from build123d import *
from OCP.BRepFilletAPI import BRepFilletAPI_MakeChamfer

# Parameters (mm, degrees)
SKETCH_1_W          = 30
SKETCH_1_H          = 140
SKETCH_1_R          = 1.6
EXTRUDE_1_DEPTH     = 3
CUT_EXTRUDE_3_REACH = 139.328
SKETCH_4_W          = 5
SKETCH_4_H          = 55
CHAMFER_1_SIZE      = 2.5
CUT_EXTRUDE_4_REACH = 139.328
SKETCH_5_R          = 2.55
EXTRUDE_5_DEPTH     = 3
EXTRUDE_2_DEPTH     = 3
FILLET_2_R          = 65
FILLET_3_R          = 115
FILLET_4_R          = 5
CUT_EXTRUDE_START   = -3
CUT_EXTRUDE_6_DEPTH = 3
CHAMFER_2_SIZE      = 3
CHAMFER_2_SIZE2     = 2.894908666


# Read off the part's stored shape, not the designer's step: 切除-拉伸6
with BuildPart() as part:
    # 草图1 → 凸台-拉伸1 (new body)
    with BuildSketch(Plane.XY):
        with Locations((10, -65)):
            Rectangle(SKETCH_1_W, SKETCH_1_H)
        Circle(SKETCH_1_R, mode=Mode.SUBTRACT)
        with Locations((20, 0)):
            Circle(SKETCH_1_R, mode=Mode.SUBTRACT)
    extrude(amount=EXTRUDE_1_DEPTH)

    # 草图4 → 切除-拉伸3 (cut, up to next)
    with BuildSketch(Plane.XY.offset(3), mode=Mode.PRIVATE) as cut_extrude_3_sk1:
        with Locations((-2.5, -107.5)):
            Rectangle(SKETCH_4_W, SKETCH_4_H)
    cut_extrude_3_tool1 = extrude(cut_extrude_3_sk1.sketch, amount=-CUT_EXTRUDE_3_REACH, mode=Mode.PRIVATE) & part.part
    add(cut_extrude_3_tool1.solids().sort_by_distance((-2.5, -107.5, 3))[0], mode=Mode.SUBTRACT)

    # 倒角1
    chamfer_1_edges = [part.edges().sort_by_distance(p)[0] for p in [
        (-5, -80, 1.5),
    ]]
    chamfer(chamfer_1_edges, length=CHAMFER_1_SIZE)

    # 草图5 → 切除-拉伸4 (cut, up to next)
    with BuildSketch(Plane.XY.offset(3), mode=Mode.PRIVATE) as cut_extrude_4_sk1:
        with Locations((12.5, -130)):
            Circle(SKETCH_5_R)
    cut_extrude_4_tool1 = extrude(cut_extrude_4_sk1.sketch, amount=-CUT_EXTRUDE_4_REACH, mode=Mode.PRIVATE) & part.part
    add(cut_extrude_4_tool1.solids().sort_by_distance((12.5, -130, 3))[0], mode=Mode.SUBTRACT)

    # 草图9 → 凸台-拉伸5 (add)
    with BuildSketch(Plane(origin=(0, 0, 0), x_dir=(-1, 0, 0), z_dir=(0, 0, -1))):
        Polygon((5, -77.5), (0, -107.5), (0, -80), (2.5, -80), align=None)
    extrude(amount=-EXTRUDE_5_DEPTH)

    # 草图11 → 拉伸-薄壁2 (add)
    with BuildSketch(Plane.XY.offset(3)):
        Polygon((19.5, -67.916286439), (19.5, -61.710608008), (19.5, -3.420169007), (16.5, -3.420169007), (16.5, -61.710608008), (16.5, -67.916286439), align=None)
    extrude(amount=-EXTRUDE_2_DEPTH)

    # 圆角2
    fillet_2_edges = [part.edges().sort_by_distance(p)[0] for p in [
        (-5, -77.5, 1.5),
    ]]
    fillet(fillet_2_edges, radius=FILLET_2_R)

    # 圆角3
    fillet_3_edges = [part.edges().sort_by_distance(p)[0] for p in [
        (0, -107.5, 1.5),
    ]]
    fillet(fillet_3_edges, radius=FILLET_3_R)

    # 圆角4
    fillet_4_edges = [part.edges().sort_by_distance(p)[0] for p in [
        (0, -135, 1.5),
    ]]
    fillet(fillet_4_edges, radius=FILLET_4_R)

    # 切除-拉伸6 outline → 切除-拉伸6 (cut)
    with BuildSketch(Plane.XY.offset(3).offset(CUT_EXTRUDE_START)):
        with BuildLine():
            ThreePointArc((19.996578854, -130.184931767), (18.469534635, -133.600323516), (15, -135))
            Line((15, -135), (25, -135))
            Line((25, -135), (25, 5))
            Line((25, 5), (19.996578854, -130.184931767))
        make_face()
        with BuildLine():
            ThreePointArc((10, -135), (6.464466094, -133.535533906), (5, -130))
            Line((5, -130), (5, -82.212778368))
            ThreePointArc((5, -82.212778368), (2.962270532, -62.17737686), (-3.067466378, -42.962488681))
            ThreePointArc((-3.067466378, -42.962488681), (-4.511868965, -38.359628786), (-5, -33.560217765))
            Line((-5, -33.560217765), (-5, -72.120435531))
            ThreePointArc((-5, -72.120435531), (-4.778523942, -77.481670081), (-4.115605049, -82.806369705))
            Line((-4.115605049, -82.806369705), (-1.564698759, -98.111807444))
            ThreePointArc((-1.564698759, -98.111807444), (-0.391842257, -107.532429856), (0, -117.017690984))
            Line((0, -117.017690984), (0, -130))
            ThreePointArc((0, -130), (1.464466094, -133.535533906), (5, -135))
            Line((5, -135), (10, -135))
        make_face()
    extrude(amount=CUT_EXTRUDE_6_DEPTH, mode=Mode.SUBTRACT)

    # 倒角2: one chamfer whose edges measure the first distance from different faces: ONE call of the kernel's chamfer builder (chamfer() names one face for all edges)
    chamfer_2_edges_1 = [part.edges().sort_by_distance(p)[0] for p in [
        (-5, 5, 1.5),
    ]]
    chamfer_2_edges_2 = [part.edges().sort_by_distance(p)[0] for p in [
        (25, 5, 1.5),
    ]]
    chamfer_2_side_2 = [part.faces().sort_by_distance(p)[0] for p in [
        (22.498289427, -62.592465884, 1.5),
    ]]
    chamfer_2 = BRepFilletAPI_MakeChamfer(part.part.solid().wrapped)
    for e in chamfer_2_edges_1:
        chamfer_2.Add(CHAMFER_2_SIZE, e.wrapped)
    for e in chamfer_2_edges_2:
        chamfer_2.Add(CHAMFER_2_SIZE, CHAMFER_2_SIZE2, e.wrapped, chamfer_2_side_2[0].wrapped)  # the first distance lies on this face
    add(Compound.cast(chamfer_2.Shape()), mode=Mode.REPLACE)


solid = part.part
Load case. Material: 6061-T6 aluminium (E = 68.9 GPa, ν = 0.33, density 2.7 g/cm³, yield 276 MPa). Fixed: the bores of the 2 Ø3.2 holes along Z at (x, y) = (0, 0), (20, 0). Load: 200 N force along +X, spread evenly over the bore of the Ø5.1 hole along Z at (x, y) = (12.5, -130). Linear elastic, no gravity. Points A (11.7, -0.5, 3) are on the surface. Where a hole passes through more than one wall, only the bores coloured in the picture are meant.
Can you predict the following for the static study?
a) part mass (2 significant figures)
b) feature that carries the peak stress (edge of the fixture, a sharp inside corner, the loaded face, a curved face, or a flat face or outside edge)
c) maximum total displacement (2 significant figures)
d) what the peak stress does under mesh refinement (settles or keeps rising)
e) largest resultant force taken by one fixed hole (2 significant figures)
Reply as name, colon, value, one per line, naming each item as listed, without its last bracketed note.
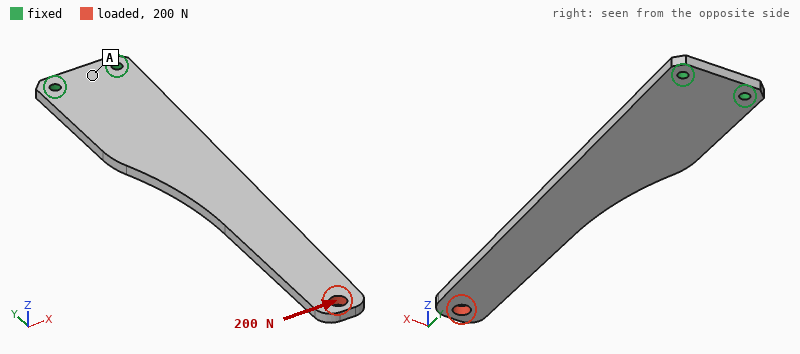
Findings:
part mass: 24 g
feature that carries the peak stress: edge of the fixture
maximum total displacement: 0.68 mm
what the peak stress does under mesh refinement: keeps rising
largest resultant force taken by one fixed hole: 1.2 kN
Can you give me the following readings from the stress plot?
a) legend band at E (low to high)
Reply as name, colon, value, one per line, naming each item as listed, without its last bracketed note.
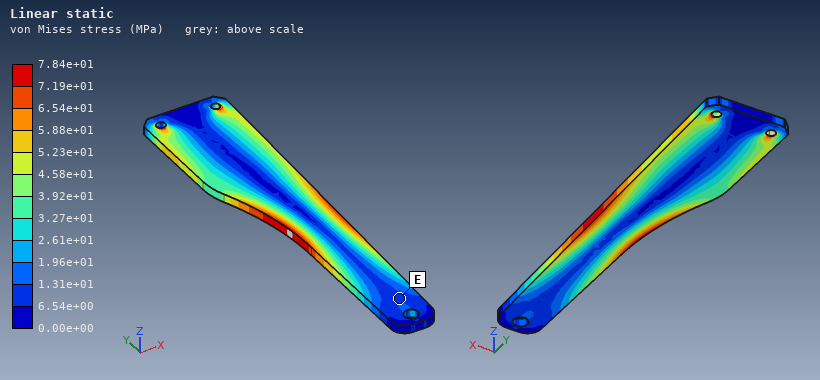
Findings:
legend band at E: 6.54e+00 to 1.31e+01 MPa
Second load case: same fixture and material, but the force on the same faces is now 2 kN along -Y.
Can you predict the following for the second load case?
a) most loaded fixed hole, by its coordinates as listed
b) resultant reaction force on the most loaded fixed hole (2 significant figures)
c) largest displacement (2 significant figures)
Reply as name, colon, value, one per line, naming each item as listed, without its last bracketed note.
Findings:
most loaded fixed hole, by its coordinates as listed: (20, 0)
resultant reaction force on the most loaded fixed hole: 1.2 kN
largest displacement: 85 µm
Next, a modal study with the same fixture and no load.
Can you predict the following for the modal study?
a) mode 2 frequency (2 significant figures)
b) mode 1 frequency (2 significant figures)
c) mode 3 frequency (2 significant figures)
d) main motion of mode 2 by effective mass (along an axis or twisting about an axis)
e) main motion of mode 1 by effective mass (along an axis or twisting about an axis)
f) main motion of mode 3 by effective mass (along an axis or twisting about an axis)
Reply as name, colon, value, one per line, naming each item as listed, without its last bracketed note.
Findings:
mode 2 frequency: 910 Hz
mode 1 frequency: 180 Hz
mode 3 frequency: 1500 Hz
main motion of mode 2 by effective mass: along Z
main motion of mode 1 by effective mass: along Z
main motion of mode 3 by effective mass: along X
